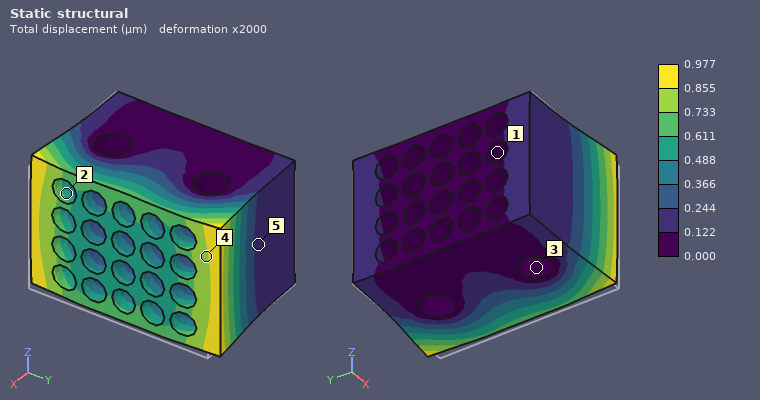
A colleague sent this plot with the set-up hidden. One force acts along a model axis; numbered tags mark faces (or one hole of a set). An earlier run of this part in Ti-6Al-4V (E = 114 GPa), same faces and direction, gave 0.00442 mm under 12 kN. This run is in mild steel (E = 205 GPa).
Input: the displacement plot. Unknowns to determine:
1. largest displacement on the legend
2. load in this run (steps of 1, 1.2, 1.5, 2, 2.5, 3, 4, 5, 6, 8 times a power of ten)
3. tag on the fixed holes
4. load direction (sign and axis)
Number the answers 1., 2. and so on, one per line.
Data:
1. 0.977 µm
2. 5 kN
3. 3
4. -X
